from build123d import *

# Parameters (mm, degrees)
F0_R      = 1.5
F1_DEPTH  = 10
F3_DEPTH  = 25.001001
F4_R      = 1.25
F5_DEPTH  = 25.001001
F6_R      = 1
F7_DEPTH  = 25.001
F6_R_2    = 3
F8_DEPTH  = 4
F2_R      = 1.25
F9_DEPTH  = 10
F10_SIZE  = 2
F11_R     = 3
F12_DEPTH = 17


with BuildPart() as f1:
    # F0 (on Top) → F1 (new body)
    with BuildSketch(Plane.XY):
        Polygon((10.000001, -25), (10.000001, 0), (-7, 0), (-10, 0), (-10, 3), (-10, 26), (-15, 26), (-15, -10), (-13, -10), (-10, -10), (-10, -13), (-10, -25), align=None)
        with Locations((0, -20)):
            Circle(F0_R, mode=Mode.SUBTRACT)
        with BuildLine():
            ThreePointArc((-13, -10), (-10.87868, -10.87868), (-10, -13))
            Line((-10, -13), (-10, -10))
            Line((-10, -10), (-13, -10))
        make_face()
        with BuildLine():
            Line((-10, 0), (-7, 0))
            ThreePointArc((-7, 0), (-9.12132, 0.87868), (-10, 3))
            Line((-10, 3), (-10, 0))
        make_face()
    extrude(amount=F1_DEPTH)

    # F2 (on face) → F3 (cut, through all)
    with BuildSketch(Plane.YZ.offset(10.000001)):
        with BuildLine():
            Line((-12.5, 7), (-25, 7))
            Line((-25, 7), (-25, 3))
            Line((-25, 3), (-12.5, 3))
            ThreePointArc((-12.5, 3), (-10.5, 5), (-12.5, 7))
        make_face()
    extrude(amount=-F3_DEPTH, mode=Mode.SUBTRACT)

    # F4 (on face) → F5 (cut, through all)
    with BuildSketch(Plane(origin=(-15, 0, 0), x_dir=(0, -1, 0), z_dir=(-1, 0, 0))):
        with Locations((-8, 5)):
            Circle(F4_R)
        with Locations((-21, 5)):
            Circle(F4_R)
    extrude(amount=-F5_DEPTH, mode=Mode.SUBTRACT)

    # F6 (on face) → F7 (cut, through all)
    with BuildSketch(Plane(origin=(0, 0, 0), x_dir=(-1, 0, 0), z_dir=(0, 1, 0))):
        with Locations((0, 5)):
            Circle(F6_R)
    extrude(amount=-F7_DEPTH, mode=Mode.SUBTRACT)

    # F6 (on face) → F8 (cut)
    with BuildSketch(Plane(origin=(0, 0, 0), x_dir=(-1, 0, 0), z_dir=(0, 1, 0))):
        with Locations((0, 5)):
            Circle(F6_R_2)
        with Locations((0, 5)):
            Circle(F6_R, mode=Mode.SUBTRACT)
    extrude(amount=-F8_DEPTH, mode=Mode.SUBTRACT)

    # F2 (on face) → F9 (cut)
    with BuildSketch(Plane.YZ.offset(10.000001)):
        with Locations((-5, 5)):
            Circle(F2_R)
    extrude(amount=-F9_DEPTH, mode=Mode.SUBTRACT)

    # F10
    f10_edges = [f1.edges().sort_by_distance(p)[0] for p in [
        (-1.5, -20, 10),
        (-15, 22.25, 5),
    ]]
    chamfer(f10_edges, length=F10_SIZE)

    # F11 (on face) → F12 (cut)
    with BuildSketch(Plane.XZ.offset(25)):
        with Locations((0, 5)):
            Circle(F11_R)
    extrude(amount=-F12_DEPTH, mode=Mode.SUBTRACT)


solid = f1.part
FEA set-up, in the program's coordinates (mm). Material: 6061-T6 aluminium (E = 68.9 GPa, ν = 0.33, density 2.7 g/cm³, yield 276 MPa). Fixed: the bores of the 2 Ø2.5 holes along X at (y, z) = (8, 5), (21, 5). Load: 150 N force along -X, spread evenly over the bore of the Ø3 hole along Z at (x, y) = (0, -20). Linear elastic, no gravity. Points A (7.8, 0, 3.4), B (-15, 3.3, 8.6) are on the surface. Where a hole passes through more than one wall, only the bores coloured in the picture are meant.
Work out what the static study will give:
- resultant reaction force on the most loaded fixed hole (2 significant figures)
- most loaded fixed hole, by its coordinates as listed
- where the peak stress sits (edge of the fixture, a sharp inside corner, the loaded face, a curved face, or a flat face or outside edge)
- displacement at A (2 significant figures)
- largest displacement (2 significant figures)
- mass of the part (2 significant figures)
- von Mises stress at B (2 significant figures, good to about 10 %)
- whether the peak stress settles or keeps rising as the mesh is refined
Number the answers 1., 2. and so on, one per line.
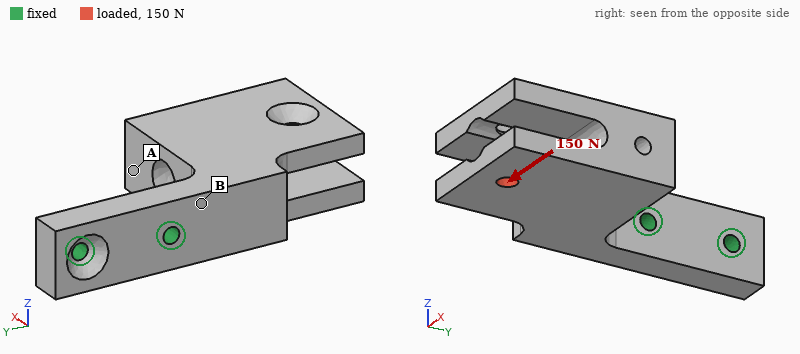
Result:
1. 210 N
2. (8, 5)
3. edge of the fixture
4. 0.096 mm
5. 0.18 mm
6. 14 g
7. 78 MPa
8. keeps rising
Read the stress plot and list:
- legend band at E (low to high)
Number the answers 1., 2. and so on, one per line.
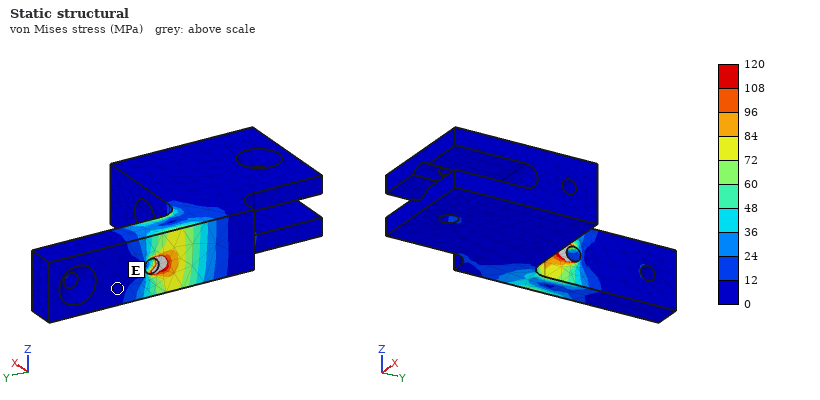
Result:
1. 0 to 12 MPa
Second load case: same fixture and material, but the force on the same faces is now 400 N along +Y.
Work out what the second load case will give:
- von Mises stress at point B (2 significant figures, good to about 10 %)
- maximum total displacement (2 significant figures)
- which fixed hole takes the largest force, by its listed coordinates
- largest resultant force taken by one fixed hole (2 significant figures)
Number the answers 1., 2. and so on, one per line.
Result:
1. 110 MPa
2. 0.24 mm
3. (8, 5)
4. 400 N
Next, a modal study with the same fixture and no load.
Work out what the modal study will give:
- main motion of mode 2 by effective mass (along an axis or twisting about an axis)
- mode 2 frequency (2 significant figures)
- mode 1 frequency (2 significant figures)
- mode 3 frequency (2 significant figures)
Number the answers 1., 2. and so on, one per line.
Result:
1. along Z
2. 2800 Hz
3. 2100 Hz
4. 6400 Hz
